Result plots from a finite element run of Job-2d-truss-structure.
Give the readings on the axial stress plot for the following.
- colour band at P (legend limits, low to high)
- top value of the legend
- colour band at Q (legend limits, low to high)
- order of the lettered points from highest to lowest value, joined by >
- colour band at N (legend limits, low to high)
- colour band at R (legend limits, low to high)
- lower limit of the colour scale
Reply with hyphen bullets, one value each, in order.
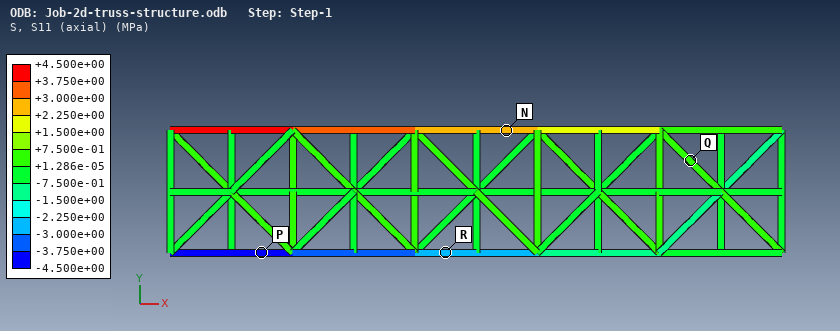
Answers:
- -4.500e+00 to -3.750e+00 MPa
- +4.500e+00 MPa
- +1.286e-05 to +7.500e-01 MPa
- N > Q > R > P
- +2.250e+00 to +3.000e+00 MPa
- -3.000e+00 to -2.250e+00 MPa
- -4.500e+00 MPa
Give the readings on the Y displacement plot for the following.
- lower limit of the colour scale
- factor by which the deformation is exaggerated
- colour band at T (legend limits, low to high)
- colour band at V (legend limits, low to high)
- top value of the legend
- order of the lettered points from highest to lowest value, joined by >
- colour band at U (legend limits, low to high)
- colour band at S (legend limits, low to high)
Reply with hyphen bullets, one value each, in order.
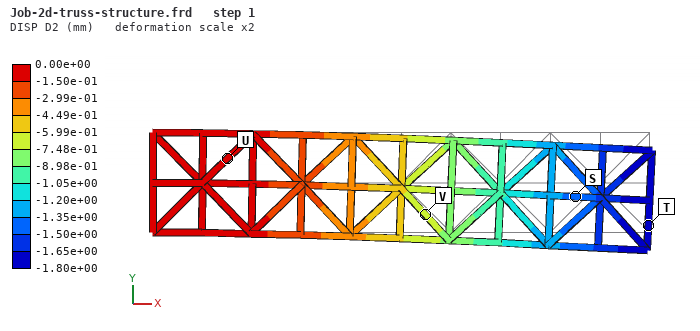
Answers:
- -1.80e+00 mm
- 2
- -1.80e+00 to -1.65e+00 mm
- -7.48e-01 to -5.99e-01 mm
- 0.00e+00 mm
- U > V > S > T
- -1.50e-01 to 0.00e+00 mm
- -1.50e+00 to -1.35e+00 mm
